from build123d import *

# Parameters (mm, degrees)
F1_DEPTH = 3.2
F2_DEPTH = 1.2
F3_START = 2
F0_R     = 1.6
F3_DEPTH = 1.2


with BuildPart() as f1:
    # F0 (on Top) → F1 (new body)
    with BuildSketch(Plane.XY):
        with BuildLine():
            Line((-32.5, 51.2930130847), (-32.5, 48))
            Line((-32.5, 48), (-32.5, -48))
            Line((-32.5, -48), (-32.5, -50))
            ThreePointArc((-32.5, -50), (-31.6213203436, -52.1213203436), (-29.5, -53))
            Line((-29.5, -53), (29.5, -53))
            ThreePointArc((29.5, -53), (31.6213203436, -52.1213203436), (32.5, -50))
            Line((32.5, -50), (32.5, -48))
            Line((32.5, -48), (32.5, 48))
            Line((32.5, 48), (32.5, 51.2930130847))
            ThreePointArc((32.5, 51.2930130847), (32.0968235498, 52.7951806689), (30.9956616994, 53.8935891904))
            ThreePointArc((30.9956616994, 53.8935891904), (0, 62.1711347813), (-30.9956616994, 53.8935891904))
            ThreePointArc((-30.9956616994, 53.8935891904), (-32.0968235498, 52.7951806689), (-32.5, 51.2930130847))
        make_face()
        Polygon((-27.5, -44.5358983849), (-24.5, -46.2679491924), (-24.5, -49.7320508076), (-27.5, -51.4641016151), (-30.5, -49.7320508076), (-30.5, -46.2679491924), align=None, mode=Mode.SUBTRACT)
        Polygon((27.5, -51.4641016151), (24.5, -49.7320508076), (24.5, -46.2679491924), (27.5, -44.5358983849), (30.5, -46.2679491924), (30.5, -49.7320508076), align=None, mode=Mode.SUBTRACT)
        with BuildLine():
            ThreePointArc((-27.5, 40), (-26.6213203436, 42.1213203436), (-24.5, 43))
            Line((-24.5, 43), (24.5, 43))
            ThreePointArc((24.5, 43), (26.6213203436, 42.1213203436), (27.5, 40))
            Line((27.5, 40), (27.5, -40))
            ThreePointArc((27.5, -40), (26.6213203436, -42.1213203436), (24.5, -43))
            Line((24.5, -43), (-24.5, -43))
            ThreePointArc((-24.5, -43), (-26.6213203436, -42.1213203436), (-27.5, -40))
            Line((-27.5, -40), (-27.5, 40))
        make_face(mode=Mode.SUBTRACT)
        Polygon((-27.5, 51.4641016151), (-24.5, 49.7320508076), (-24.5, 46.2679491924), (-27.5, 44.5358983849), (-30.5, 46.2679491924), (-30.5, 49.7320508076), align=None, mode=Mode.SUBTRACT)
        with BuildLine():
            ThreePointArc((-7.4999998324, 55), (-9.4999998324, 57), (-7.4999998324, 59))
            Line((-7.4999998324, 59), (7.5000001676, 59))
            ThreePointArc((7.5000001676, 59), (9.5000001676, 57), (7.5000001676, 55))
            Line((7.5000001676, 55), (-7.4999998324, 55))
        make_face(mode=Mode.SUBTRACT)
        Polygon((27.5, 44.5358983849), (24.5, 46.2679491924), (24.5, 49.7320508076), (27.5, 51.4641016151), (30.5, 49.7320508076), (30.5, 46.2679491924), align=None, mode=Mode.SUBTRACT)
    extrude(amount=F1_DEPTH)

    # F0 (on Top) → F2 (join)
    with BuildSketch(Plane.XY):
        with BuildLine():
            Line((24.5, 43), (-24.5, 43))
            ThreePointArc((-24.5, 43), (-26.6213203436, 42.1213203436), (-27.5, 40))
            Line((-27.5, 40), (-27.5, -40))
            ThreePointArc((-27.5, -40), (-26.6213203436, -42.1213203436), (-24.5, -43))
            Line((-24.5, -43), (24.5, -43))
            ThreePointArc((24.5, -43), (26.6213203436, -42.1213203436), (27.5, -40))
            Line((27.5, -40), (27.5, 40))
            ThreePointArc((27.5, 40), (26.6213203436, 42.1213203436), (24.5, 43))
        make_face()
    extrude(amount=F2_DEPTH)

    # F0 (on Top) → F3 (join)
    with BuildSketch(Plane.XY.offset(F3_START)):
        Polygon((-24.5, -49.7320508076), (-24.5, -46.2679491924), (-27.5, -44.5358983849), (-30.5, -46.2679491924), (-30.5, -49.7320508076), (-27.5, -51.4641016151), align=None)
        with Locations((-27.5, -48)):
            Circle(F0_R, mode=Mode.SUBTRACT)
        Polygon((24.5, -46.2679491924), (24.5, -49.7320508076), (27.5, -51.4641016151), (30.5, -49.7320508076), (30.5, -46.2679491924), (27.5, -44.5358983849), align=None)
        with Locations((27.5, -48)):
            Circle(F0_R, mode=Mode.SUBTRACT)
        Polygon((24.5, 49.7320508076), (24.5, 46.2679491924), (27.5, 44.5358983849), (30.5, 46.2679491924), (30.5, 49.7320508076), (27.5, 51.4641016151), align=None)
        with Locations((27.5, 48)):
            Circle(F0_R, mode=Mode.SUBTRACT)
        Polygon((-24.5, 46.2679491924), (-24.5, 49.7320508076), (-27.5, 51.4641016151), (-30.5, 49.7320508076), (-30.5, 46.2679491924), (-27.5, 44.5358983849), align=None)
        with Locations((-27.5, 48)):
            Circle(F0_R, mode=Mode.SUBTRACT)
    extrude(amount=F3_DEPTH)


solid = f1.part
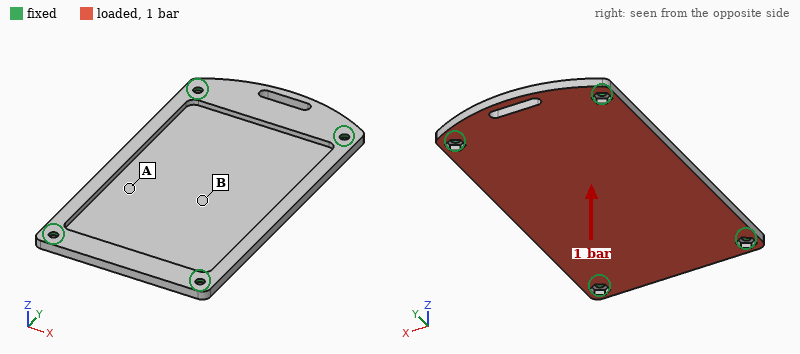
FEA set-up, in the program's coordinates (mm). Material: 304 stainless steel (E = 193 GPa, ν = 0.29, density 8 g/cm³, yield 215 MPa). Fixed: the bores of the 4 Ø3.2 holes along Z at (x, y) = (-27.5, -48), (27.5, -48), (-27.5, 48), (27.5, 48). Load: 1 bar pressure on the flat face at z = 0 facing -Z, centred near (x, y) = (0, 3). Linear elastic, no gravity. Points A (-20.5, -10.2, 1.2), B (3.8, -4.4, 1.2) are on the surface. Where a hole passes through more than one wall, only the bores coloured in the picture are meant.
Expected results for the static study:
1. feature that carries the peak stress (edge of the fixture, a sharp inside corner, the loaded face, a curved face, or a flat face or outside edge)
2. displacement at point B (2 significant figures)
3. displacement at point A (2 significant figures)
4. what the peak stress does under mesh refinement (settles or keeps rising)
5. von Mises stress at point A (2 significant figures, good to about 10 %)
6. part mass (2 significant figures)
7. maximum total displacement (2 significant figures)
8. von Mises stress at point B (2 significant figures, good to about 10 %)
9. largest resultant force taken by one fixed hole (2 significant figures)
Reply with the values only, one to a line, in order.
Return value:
edge of the fixture
0.26 mm
0.18 mm
keeps rising
19 MPa
110 g
0.26 mm
49 MPa
690 N
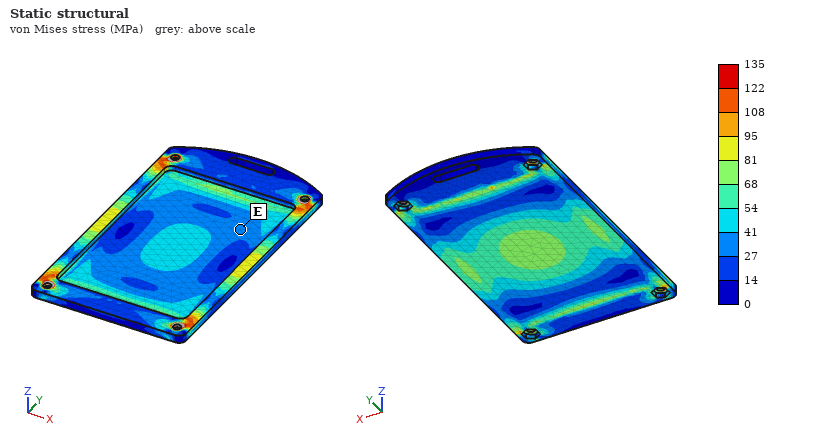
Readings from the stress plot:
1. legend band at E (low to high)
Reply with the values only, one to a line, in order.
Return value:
27 to 41 MPa
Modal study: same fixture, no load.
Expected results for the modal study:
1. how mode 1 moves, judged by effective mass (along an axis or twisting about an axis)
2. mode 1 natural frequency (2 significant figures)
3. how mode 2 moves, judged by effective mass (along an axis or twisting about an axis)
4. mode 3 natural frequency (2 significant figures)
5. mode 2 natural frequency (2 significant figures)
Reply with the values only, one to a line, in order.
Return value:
along Z
1200 Hz
twisting about Y
2500 Hz
1600 Hz
